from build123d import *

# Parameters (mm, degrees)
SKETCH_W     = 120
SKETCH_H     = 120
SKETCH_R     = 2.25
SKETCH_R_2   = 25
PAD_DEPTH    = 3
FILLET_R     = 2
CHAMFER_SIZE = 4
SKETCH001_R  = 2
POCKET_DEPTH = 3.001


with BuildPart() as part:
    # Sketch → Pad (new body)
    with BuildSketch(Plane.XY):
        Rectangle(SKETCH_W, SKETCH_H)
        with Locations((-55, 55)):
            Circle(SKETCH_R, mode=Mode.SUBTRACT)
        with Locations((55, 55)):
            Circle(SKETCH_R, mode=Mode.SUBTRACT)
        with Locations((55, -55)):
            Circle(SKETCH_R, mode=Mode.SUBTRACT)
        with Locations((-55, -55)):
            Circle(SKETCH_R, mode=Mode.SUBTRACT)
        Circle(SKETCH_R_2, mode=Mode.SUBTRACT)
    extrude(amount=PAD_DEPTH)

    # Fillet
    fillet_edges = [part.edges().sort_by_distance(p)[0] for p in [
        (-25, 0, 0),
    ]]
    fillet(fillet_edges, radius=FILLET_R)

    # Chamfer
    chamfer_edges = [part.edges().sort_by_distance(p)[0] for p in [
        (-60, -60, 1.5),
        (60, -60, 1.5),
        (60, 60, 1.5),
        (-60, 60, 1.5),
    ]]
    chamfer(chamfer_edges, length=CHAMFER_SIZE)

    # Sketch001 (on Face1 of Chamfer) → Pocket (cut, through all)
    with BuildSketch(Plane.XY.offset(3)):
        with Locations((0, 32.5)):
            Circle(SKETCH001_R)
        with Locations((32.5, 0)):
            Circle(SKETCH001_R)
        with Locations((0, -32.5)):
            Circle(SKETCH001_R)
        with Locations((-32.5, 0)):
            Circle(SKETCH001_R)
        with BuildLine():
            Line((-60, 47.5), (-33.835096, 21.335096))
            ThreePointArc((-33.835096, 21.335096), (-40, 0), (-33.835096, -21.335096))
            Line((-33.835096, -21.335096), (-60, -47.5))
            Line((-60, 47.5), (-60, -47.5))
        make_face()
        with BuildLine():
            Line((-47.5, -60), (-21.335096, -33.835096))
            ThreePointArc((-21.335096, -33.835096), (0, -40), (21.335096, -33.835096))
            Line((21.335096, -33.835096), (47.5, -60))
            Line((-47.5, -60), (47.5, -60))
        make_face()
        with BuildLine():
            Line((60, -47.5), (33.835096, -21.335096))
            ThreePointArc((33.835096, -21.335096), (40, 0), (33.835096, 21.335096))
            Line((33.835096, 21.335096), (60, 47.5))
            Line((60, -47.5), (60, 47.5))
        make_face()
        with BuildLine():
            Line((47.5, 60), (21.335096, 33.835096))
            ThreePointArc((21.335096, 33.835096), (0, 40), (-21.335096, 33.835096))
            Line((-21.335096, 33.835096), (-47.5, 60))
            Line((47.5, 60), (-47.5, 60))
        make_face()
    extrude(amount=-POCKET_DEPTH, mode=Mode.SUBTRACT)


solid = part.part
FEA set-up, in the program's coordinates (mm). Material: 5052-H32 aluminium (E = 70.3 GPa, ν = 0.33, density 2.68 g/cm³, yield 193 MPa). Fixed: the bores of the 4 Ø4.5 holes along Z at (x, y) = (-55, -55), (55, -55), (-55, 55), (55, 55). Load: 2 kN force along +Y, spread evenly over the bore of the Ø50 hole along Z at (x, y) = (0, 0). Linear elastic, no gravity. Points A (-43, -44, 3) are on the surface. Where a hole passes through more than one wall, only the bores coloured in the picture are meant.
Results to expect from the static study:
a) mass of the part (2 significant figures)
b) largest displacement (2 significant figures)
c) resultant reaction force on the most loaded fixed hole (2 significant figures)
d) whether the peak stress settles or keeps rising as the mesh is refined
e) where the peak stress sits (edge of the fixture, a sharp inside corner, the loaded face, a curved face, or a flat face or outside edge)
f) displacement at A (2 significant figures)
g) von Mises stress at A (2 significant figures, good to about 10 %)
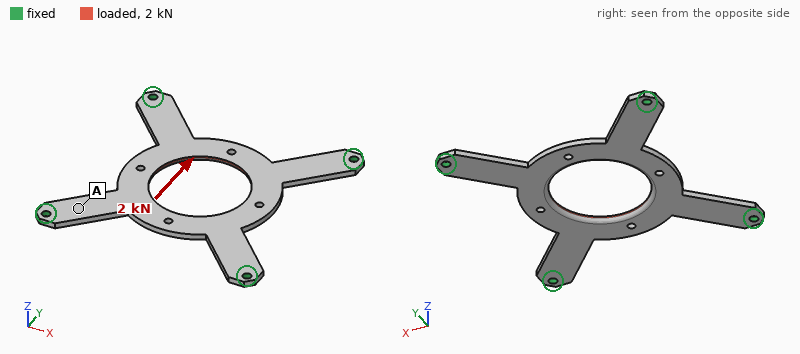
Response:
46 g
52 µm
670 N
keeps rising
edge of the fixture
9.5 µm
13 MPa
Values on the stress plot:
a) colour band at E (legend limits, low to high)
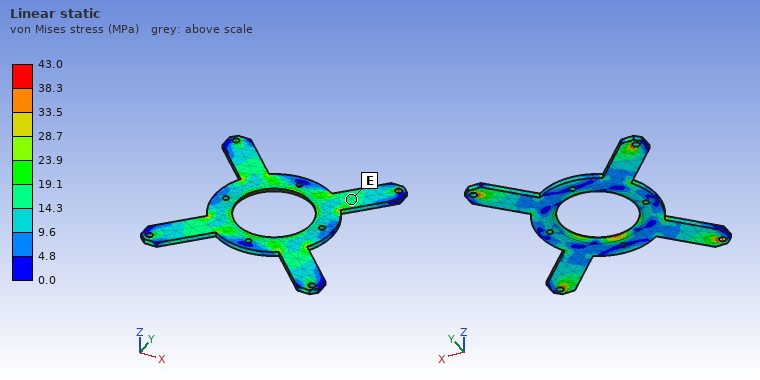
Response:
14.3 to 19.1 MPa
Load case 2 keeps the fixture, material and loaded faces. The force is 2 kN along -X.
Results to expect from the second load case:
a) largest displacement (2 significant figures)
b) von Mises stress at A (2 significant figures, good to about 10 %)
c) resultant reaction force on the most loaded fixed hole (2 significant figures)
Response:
52 µm
13 MPa
670 N
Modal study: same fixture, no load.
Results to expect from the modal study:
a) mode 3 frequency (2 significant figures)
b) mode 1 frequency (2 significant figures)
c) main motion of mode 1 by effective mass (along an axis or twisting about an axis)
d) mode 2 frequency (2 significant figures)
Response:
1500 Hz
810 Hz
along Z
1500 Hz
